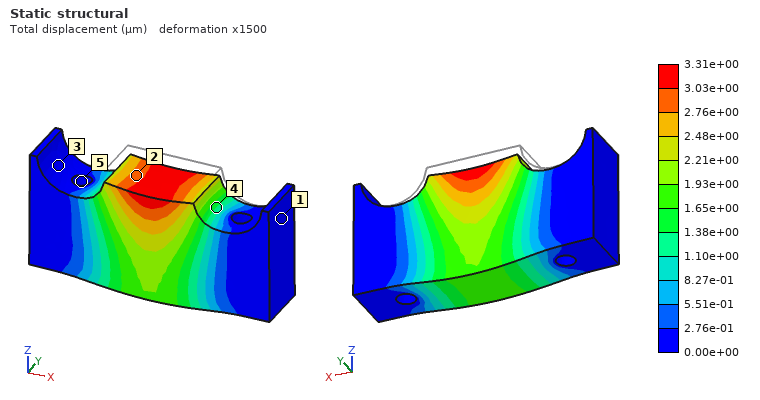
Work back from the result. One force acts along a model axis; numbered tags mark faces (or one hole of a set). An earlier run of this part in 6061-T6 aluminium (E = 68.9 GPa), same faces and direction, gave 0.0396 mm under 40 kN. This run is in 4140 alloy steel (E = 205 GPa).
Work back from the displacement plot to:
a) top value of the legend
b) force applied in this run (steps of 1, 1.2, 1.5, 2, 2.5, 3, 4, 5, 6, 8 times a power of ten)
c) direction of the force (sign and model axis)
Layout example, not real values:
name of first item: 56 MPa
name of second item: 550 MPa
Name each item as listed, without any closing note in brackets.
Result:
top value of the legend: 3.31e+00 µm
force applied in this run: 10 kN
direction of the force: -Z
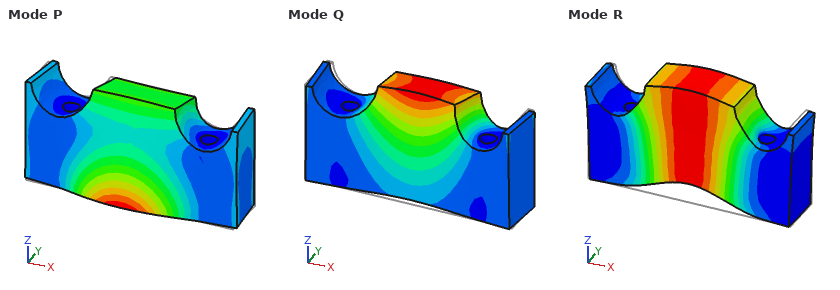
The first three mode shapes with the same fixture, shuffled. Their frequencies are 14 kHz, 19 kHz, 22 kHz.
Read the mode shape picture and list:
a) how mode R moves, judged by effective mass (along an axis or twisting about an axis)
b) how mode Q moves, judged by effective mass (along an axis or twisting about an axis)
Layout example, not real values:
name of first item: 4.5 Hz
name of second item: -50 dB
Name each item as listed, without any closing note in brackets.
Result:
how mode R moves, judged by effective mass: along Z
how mode Q moves, judged by effective mass: along Y
